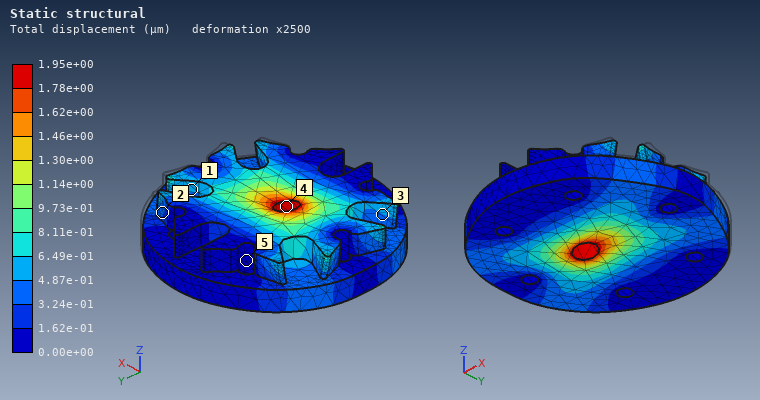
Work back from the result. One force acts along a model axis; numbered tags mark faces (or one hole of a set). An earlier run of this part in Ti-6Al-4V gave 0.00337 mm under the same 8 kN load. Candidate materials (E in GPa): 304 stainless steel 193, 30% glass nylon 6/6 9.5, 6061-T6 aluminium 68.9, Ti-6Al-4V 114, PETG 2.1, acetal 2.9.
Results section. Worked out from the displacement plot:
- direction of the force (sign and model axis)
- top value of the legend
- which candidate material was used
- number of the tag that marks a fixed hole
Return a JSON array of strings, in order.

["-X", "1.95e+00 µm", "304 stainless steel", "5"]
